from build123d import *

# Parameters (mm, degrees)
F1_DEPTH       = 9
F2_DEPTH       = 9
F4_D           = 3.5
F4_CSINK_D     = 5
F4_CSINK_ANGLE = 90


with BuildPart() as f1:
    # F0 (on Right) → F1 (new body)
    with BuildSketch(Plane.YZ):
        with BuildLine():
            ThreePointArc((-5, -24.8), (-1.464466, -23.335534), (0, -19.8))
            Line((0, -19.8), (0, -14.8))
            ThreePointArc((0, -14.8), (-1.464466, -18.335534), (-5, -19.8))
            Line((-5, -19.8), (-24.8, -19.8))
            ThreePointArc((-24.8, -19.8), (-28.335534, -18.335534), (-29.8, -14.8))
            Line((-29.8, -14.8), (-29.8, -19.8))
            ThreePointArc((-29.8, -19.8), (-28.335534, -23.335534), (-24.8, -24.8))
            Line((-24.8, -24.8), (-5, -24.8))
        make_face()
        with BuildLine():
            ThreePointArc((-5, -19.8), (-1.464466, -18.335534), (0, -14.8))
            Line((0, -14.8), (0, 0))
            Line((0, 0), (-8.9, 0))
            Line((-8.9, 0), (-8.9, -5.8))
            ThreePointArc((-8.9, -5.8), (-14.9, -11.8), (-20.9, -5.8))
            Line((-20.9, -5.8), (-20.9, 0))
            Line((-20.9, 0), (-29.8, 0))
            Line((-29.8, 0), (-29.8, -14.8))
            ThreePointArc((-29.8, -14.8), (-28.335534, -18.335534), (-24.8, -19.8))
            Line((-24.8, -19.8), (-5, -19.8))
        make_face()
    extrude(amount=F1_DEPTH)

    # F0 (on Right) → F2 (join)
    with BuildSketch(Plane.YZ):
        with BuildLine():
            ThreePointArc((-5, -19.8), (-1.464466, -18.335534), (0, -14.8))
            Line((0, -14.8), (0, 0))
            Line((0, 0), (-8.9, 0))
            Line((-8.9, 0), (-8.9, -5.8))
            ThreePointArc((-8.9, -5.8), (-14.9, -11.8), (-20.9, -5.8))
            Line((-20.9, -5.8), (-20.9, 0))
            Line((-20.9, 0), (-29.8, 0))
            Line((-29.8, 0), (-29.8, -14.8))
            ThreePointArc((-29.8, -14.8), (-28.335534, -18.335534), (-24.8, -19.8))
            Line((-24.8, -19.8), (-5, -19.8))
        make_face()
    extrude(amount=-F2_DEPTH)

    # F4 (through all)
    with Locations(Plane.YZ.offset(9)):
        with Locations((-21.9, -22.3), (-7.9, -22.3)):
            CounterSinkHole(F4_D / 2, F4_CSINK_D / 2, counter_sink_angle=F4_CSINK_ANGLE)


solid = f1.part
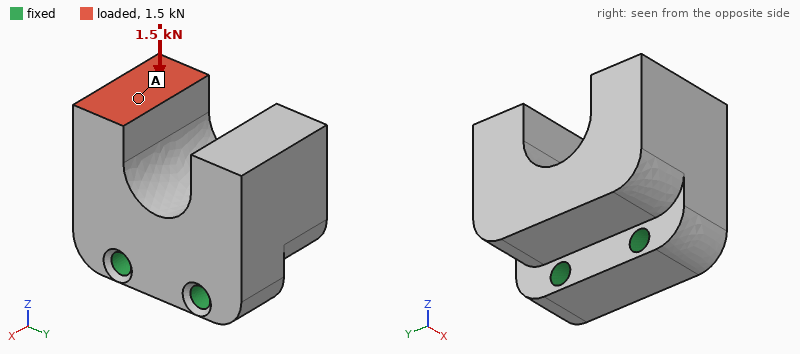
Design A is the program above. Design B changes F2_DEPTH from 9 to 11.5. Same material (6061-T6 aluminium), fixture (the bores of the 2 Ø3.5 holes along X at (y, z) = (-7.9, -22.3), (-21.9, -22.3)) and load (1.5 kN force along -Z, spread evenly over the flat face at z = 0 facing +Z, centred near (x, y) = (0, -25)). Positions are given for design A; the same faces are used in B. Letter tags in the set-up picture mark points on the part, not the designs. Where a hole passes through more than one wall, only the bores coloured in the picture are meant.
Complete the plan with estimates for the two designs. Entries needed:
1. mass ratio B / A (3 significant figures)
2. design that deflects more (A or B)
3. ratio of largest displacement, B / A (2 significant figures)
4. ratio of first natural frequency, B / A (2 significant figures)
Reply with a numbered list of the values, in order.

1. 1.12
2. B
3. 1.2
4. 0.88
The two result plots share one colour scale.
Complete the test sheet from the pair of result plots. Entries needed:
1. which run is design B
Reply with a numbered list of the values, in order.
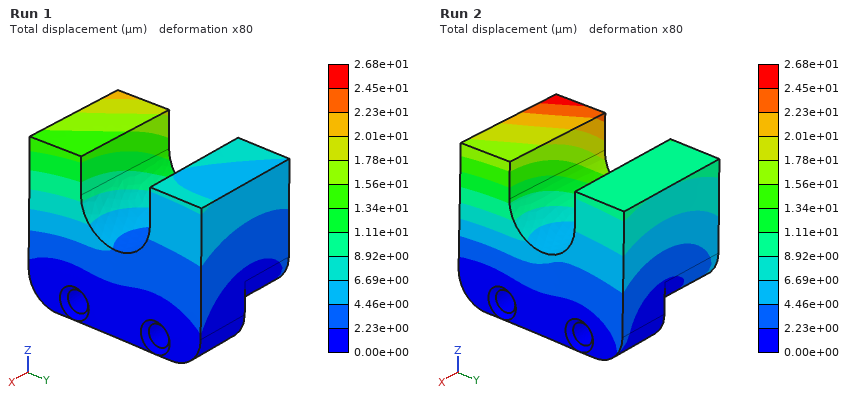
1. Run 2
